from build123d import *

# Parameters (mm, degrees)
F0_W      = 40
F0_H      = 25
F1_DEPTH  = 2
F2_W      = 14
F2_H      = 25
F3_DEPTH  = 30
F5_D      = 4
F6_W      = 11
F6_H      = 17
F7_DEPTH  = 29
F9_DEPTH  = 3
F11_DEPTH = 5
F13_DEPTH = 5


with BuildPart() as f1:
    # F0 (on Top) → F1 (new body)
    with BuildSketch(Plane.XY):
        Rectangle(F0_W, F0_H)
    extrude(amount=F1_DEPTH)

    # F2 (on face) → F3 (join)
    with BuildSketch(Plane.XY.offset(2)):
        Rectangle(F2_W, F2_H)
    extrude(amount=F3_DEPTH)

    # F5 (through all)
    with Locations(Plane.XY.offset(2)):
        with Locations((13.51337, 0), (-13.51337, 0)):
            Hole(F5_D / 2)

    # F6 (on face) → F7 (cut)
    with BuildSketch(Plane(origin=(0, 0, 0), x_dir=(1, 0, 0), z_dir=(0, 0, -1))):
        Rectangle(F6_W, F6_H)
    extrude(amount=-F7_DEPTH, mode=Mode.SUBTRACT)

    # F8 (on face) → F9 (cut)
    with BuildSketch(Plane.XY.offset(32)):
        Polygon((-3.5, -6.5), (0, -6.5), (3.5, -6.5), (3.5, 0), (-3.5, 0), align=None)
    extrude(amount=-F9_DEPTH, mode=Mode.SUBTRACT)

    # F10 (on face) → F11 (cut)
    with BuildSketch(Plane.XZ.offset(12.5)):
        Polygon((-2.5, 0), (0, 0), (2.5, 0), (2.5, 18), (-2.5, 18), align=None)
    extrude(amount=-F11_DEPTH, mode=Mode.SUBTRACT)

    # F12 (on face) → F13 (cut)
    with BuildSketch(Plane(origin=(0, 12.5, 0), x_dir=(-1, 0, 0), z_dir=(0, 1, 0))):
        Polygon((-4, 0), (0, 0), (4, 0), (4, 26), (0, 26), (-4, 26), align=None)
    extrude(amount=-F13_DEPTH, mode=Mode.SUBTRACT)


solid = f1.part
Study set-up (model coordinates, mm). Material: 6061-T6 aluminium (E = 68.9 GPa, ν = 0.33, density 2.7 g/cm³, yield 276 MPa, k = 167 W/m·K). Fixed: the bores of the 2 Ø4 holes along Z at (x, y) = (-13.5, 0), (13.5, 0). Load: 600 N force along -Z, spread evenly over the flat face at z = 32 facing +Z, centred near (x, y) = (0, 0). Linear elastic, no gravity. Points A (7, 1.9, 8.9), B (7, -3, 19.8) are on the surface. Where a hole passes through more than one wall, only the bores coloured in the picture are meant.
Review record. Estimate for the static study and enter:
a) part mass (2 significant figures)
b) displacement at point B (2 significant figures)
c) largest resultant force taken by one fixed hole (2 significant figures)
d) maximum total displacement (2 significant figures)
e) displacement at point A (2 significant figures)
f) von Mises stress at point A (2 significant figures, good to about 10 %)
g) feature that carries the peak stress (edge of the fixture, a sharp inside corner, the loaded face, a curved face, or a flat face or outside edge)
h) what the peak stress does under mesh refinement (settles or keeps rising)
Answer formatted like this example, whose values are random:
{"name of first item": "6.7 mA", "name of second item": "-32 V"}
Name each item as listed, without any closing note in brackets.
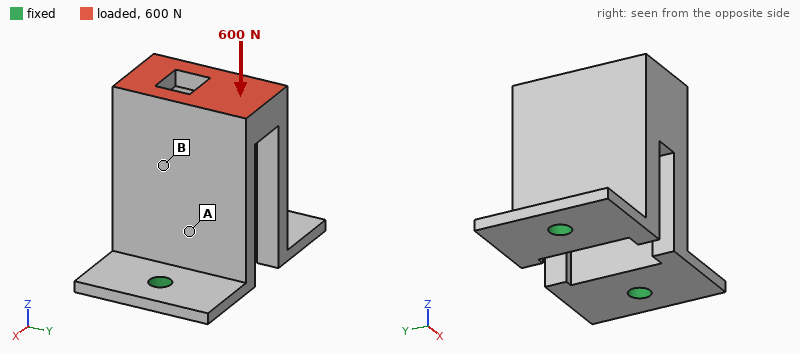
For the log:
{"part mass": "15 g", "displacement at point B": "26 µm", "largest resultant force taken by one fixed hole": "300 N", "maximum total displacement": "40 µm", "displacement at point A": "28 µm", "von Mises stress at point A": "22 MPa", "feature that carries the peak stress": "edge of the fixture", "what the peak stress does under mesh refinement": "keeps rising"}
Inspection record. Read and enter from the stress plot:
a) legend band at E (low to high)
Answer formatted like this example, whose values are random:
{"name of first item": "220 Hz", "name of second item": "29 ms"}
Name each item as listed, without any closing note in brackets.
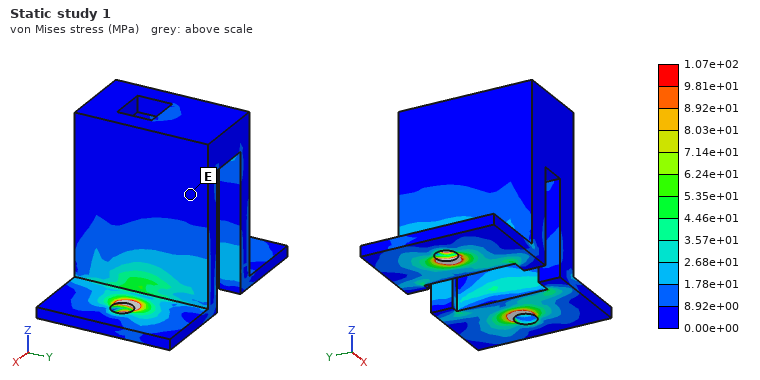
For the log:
{"legend band at E": "0.00e+00 to 8.92e+00 MPa"}
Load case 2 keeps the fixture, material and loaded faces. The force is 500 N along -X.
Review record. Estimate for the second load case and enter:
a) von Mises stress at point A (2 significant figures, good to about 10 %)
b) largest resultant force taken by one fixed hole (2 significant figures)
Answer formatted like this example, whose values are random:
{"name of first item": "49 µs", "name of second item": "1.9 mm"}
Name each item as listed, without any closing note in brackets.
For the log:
{"von Mises stress at point A": "67 MPa", "largest resultant force taken by one fixed hole": "820 N"}
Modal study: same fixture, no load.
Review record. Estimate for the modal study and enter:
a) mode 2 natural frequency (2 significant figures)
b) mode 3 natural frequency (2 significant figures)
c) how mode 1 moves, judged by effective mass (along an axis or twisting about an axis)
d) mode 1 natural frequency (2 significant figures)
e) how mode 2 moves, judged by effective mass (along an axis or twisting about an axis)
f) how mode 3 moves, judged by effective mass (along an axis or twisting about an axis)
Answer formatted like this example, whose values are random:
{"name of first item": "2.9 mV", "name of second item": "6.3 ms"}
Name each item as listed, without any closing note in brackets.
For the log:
{"mode 2 natural frequency": "2800 Hz", "mode 3 natural frequency": "5700 Hz", "how mode 1 moves, judged by effective mass": "along Y", "mode 1 natural frequency": "1700 Hz", "how mode 2 moves, judged by effective mass": "along X", "how mode 3 moves, judged by effective mass": "twisting about Z"}
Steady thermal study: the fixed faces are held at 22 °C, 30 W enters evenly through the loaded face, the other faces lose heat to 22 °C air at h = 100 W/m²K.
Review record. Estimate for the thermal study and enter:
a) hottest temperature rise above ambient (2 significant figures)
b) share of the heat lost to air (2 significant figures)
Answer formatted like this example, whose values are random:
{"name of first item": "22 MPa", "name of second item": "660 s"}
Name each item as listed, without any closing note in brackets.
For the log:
{"hottest temperature rise above ambient": "49 K", "share of the heat lost to air": "41 %"}
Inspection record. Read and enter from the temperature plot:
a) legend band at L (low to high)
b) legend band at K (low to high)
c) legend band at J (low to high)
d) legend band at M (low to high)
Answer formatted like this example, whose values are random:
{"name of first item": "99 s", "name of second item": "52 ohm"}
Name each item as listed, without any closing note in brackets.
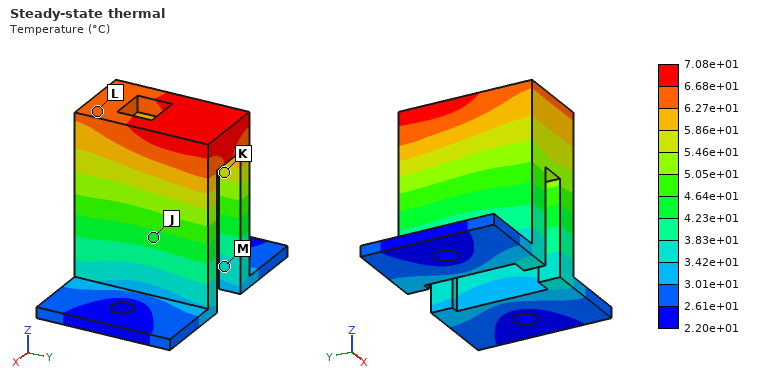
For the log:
{"legend band at L": "6.27e+01 to 6.68e+01 °C", "legend band at K": "5.46e+01 to 5.86e+01 °C", "legend band at J": "4.23e+01 to 4.64e+01 °C", "legend band at M": "3.42e+01 to 3.83e+01 °C"}
